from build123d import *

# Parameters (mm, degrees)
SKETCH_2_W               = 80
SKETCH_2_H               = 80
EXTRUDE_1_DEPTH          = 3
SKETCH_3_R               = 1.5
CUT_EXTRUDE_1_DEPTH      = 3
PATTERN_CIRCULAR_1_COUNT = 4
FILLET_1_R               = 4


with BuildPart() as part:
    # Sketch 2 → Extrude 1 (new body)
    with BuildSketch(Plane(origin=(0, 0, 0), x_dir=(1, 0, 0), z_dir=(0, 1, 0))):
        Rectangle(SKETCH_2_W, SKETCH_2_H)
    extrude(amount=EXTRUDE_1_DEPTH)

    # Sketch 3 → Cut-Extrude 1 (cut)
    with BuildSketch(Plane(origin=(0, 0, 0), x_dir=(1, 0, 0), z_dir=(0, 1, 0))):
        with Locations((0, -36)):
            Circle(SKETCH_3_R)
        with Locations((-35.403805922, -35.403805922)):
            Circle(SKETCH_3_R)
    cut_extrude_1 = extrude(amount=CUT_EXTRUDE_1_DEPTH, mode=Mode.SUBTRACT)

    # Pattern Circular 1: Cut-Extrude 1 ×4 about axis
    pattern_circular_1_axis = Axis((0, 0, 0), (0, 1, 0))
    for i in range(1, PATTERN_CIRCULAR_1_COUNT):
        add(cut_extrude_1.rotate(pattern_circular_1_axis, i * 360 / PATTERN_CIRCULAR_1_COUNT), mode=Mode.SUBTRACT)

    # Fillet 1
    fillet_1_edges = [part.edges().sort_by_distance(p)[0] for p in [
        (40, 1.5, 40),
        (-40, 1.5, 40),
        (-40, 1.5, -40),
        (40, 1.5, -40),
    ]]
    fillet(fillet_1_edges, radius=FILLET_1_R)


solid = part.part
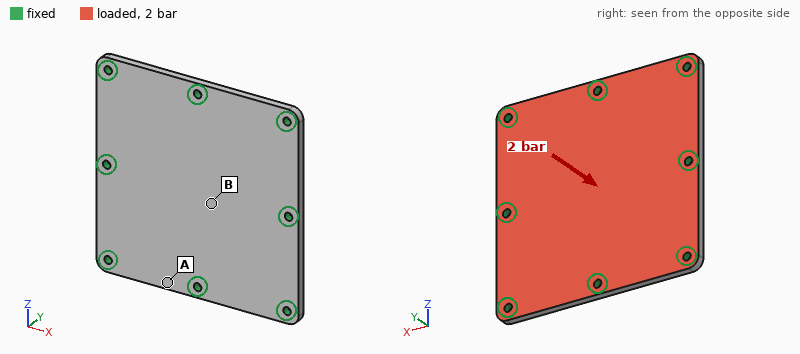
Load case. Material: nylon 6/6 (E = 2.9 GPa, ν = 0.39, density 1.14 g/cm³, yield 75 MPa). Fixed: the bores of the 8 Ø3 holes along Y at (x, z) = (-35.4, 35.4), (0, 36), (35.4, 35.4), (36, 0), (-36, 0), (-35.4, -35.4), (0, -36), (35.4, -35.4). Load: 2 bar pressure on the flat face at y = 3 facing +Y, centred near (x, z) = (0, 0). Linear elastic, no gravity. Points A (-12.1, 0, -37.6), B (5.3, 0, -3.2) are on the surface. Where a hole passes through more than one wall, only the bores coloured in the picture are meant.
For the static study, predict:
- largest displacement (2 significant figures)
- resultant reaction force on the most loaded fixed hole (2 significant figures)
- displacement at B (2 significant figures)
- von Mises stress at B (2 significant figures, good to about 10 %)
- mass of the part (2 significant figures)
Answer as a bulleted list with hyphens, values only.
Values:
- 1.3 mm
- 230 N
- 1.2 mm
- 19 MPa
- 22 g
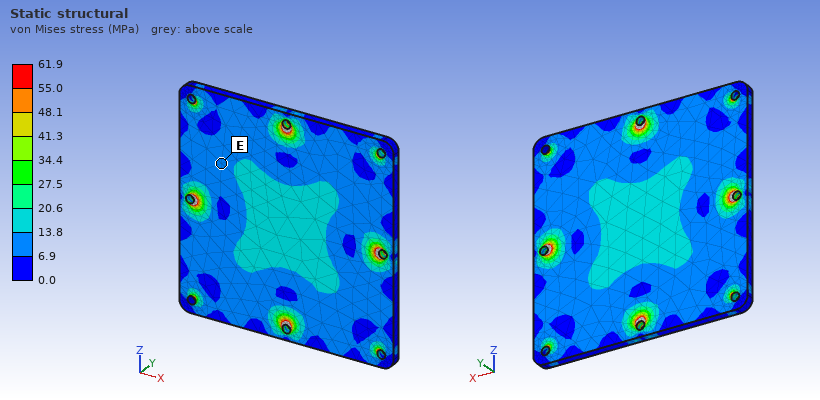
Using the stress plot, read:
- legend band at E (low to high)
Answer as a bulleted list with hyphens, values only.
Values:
- 6.9 to 13.8 MPa
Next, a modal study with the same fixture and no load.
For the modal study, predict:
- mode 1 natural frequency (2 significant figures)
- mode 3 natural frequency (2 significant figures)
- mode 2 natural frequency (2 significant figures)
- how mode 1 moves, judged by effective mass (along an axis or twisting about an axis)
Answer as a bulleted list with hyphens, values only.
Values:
- 1400 Hz
- 2500 Hz
- 2500 Hz
- along Y
